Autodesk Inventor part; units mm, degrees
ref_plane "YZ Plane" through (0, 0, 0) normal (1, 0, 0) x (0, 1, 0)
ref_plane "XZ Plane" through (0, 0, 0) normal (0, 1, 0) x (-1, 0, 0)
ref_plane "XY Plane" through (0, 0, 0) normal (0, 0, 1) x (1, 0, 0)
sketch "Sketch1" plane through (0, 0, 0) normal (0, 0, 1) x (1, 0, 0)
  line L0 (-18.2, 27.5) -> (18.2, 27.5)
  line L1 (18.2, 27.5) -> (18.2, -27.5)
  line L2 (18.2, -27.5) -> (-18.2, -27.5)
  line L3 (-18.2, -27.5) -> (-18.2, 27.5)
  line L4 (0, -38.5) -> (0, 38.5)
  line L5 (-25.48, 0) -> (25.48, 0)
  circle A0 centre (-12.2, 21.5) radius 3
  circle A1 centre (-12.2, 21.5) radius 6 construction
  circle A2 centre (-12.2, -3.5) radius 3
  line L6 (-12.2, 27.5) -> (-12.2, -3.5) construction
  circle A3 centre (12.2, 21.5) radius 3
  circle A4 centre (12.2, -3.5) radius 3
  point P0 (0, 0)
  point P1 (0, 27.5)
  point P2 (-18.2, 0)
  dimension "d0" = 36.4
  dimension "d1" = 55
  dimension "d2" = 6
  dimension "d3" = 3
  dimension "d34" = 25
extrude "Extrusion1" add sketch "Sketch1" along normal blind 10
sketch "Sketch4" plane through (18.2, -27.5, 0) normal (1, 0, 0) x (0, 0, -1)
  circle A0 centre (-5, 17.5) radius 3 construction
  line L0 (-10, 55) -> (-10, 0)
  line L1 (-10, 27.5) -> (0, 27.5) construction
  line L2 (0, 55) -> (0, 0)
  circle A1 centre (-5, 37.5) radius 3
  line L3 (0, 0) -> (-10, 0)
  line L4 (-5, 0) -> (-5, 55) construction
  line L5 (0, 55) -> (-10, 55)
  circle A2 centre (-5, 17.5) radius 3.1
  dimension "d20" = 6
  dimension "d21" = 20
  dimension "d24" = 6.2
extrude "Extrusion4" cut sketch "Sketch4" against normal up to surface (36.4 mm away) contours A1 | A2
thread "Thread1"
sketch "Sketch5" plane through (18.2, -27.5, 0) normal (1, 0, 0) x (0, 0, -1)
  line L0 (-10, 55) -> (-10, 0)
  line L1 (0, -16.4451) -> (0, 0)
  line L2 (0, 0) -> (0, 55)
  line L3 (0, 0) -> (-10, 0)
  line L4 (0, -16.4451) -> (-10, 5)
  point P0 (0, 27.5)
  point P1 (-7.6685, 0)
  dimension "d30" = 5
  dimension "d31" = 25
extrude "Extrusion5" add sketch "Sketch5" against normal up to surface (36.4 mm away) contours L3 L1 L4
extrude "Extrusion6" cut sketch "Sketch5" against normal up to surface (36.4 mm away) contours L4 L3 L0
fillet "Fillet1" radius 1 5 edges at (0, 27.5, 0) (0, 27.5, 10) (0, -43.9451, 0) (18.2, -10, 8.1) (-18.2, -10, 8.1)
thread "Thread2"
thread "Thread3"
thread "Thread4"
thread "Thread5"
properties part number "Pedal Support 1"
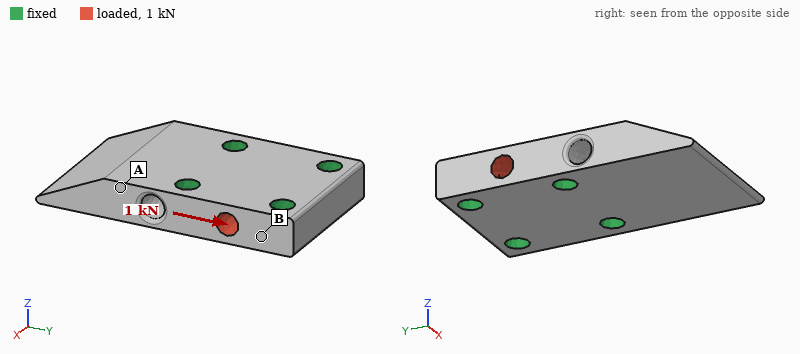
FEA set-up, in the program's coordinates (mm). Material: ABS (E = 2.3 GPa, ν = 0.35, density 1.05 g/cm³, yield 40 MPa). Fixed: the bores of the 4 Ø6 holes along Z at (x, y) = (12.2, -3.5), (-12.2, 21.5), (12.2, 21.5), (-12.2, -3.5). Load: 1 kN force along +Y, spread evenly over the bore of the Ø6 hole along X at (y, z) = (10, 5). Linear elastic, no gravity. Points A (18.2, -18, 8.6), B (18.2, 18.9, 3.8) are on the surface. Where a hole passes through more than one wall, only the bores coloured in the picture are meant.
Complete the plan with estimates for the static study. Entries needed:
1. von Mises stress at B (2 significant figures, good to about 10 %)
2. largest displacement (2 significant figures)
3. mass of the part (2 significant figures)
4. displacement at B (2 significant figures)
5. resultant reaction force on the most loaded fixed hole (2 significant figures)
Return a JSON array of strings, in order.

["0.79 MPa", "11 µm", "20 g", "2.4 µm", "260 N"]
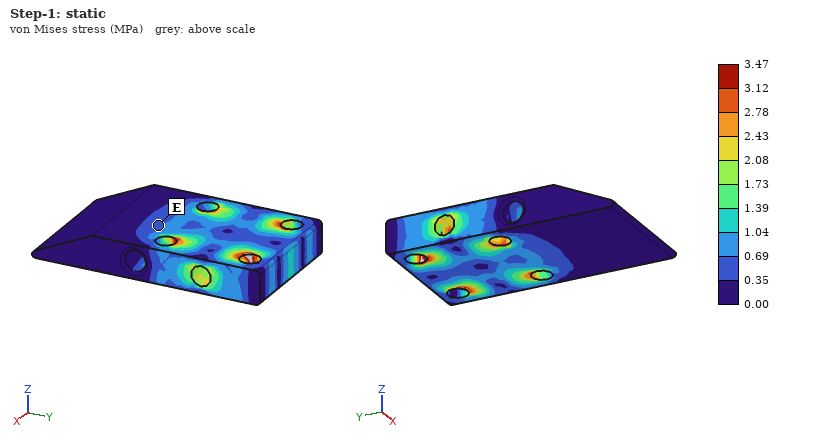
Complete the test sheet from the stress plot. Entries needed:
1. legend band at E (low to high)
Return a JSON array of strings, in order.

["0.35 to 0.69 MPa"]
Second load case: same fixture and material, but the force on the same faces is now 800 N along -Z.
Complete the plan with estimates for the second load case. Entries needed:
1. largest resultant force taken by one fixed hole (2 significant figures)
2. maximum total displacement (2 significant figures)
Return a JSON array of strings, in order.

["210 N", "30 µm"]
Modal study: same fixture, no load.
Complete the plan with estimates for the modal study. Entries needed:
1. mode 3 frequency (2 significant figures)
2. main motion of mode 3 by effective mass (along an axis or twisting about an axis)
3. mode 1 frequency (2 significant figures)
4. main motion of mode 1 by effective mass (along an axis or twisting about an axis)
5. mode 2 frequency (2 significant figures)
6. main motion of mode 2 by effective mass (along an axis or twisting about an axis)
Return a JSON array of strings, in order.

["4400 Hz", "along X", "2100 Hz", "along Z", "3700 Hz", "twisting about Y"]
